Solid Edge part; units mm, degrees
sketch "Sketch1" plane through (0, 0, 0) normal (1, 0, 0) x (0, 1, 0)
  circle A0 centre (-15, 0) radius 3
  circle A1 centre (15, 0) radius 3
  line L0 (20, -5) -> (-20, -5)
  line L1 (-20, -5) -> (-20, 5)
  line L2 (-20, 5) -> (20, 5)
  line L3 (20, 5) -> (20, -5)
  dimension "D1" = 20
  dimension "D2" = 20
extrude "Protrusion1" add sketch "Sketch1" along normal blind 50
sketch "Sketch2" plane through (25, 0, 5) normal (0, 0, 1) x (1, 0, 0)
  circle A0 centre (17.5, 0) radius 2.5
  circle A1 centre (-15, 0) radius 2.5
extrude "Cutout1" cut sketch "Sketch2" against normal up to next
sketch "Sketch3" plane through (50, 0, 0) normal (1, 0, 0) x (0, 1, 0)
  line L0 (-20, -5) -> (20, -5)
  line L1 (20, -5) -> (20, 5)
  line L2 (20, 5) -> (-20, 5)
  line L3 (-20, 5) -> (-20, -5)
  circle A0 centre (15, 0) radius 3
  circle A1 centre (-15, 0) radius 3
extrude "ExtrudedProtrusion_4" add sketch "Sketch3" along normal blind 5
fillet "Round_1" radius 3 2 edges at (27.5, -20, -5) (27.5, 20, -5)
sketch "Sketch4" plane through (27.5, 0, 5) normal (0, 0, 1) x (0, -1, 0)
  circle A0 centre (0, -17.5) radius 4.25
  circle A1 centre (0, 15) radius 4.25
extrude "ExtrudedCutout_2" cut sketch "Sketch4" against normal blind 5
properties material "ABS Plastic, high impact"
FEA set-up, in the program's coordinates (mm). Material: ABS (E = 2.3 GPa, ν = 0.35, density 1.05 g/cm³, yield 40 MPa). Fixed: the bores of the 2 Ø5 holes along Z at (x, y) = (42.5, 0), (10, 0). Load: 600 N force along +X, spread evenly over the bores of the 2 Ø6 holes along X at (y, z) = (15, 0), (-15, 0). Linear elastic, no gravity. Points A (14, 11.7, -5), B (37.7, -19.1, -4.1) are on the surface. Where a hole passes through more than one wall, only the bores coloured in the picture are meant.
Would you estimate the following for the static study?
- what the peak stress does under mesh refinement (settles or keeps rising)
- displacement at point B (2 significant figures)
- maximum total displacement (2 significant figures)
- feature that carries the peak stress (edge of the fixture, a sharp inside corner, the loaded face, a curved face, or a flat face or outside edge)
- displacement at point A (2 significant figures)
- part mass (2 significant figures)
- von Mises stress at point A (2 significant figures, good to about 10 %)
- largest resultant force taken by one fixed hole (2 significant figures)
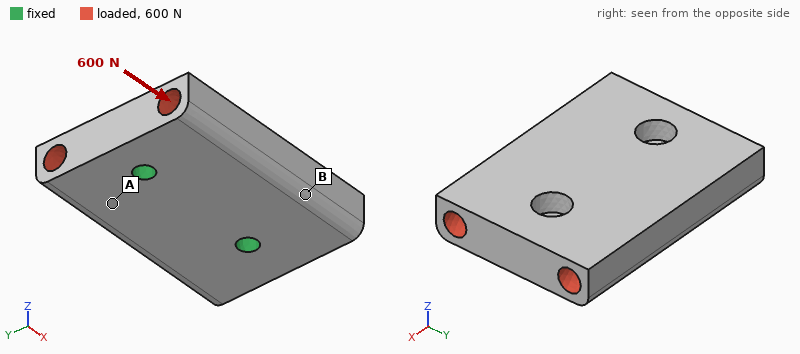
keeps rising
20 µm
28 µm
edge of the fixture
14 µm
19 g
1.3 MPa
310 N
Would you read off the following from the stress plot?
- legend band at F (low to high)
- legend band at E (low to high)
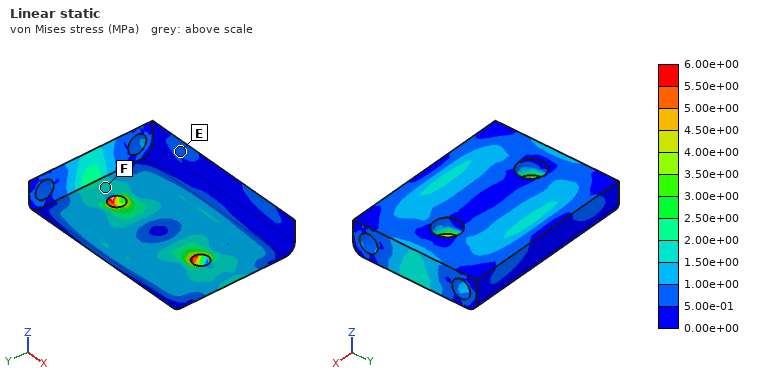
1.50e+00 to 2.00e+00 MPa
5.00e-01 to 1.00e+00 MPa
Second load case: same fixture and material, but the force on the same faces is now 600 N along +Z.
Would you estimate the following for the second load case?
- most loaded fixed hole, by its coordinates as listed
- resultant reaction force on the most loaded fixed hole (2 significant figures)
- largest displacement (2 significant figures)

(42.5, 0)
320 N
96 µm
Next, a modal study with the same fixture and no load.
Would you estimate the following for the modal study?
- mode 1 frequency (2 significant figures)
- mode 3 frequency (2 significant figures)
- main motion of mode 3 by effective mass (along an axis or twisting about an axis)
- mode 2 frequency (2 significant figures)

2300 Hz
4700 Hz
along Z
4500 Hz
